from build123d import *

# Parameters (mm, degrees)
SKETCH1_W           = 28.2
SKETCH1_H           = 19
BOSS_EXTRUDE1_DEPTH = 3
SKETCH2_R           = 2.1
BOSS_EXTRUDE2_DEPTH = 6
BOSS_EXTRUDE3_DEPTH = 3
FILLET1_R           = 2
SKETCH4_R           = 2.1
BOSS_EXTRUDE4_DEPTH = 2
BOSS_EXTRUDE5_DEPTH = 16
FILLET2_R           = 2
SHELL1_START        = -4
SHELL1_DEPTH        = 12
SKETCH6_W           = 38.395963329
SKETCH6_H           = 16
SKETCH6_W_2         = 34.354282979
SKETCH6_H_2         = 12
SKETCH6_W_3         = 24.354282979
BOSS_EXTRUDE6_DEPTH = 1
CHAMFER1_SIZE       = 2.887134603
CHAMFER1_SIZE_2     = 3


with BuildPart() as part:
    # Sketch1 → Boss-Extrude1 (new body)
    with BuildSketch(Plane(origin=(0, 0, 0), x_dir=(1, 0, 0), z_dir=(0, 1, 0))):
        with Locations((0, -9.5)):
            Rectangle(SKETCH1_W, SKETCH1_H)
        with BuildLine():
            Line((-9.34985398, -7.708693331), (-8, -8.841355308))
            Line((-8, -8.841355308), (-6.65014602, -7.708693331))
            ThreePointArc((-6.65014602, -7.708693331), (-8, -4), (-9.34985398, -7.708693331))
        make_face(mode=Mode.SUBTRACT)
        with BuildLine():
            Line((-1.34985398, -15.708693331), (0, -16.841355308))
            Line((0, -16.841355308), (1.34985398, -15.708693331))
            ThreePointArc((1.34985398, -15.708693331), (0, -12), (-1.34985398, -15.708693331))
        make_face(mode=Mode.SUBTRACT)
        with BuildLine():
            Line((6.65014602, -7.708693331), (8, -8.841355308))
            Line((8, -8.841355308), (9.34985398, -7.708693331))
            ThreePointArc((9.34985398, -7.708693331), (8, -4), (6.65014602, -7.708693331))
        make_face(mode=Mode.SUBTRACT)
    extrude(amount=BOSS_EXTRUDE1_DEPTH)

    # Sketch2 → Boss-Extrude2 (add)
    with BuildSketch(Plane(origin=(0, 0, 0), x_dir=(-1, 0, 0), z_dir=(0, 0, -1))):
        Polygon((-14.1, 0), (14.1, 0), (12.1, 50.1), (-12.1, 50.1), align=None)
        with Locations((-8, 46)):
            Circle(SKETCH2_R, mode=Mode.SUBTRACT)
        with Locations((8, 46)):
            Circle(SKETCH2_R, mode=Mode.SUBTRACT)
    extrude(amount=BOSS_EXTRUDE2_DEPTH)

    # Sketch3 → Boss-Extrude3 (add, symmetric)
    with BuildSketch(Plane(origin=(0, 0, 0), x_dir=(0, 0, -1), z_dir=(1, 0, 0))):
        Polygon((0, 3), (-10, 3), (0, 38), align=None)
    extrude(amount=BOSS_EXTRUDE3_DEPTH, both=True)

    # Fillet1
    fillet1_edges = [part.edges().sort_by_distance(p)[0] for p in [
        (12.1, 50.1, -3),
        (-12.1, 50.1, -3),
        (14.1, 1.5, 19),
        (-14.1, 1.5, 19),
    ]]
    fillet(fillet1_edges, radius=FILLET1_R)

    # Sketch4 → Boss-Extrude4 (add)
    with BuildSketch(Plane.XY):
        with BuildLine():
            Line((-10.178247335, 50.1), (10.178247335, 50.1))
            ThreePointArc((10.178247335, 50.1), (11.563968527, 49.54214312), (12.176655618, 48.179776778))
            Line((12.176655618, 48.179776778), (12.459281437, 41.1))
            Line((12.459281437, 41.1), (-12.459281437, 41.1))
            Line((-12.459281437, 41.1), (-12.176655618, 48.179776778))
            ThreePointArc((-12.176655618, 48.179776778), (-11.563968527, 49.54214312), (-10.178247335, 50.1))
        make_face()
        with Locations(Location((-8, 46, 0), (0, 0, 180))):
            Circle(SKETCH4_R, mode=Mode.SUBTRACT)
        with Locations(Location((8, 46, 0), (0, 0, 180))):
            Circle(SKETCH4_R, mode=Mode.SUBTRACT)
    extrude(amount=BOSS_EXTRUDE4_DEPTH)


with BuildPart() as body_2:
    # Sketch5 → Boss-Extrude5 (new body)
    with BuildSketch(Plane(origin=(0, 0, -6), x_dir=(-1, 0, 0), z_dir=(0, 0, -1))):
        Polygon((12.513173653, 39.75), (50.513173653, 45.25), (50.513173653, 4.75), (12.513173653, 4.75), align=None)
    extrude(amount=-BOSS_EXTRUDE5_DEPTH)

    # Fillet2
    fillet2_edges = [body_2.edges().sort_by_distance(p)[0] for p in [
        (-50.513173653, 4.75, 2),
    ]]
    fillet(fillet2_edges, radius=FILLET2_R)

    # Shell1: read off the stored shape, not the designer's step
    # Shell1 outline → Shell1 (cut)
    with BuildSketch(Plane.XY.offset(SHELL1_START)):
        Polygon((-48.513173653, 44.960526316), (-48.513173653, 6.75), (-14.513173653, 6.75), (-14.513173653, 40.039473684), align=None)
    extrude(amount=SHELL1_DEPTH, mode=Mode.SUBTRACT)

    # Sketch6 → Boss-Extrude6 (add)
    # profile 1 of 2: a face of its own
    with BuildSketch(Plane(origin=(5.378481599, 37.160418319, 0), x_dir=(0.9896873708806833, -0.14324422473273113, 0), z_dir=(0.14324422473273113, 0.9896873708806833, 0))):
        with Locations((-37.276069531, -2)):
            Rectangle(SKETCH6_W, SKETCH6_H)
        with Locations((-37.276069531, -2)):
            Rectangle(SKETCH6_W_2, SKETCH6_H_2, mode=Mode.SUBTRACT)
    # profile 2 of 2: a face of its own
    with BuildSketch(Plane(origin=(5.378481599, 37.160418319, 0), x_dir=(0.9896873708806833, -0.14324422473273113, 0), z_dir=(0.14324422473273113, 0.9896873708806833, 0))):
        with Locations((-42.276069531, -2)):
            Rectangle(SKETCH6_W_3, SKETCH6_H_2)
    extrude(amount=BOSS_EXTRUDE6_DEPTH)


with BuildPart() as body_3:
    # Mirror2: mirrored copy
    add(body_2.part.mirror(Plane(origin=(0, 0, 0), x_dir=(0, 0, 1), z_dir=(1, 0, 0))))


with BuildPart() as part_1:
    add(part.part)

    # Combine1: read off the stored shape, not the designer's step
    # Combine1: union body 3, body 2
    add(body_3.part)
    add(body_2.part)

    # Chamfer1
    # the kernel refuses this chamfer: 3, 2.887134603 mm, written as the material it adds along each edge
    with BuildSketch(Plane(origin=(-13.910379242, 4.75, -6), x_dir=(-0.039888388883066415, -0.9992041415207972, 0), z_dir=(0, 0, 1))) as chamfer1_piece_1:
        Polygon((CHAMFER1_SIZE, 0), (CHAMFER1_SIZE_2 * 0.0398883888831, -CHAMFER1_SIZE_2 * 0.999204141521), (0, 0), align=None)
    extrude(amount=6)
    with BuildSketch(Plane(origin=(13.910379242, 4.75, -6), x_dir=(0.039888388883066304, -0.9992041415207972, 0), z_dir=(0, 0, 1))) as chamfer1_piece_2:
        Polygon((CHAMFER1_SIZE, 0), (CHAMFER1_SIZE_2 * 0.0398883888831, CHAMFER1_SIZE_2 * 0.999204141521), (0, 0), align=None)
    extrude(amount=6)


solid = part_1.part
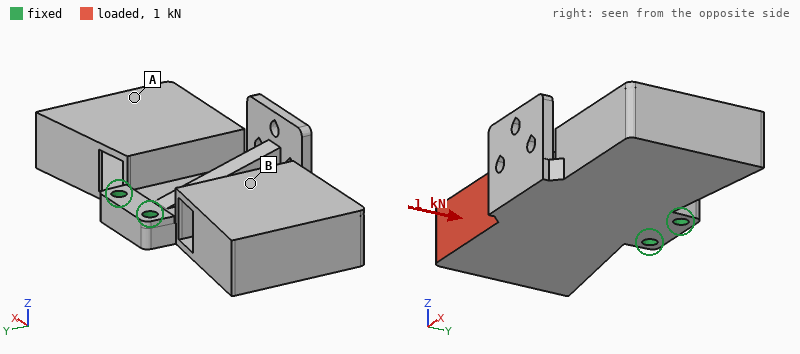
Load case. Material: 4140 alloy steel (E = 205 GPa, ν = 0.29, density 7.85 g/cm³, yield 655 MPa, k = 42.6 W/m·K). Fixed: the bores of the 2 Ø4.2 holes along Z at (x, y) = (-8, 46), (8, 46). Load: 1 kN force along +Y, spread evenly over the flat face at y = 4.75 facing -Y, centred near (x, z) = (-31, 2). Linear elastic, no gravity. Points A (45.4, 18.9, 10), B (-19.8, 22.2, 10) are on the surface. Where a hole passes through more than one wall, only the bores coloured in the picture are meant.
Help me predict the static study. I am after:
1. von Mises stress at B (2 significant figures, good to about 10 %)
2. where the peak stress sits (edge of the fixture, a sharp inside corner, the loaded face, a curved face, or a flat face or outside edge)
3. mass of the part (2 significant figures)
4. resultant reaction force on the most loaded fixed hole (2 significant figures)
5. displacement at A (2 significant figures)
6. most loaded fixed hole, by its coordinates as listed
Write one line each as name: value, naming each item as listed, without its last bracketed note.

von Mises stress at B: 12 MPa
where the peak stress sits: a flat face or outside edge
mass of the part: 220 g
resultant reaction force on the most loaded fixed hole: 2.3 kN
displacement at A: 7.4 µm
most loaded fixed hole, by its coordinates as listed: (-8, 46)
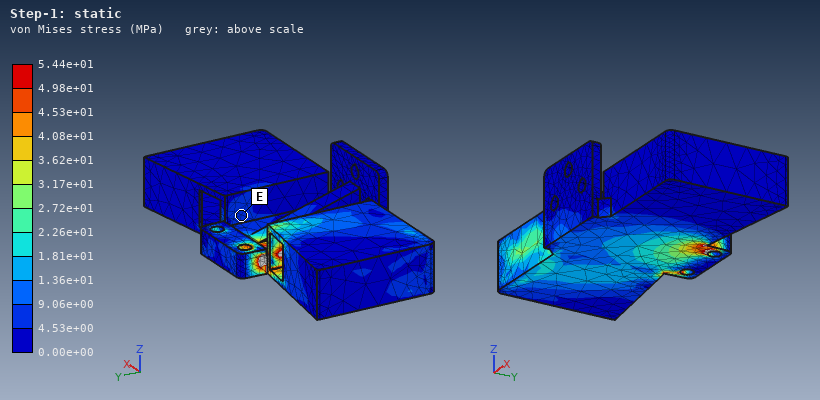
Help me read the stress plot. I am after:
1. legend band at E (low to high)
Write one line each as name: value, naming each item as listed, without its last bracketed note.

legend band at E: 4.53e+00 to 9.06e+00 MPa
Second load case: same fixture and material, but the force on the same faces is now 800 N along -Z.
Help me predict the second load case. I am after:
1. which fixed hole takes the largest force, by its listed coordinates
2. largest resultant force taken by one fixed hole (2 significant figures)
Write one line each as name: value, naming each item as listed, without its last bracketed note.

which fixed hole takes the largest force, by its listed coordinates: (-8, 46)
largest resultant force taken by one fixed hole: 1.5 kN
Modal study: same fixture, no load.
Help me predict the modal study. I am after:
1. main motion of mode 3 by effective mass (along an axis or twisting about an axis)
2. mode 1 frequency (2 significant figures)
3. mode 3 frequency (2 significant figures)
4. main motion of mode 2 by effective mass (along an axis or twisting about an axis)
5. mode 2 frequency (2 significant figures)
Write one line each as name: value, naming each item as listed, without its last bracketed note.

main motion of mode 3 by effective mass: twisting about X
mode 1 frequency: 1200 Hz
mode 3 frequency: 2100 Hz
main motion of mode 2 by effective mass: along Z
mode 2 frequency: 1300 Hz
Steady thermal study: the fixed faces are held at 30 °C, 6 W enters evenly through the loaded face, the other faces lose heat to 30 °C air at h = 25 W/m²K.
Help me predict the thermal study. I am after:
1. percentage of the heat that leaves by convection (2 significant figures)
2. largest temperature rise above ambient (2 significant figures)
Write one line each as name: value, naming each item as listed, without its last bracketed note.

percentage of the heat that leaves by convection: 63 %
largest temperature rise above ambient: 24 K
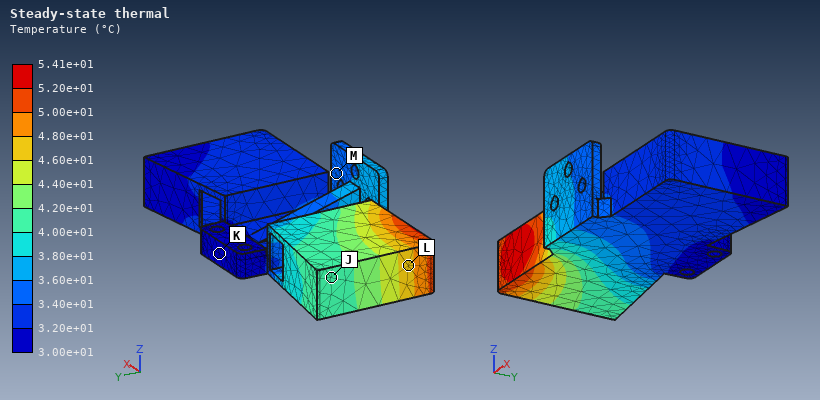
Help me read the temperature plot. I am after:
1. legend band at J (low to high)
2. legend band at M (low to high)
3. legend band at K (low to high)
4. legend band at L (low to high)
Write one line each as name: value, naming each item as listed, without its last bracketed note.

legend band at J: 4.00e+01 to 4.20e+01 °C
legend band at M: 3.40e+01 to 3.60e+01 °C
legend band at K: 3.00e+01 to 3.20e+01 °C
legend band at L: 4.60e+01 to 4.80e+01 °C
